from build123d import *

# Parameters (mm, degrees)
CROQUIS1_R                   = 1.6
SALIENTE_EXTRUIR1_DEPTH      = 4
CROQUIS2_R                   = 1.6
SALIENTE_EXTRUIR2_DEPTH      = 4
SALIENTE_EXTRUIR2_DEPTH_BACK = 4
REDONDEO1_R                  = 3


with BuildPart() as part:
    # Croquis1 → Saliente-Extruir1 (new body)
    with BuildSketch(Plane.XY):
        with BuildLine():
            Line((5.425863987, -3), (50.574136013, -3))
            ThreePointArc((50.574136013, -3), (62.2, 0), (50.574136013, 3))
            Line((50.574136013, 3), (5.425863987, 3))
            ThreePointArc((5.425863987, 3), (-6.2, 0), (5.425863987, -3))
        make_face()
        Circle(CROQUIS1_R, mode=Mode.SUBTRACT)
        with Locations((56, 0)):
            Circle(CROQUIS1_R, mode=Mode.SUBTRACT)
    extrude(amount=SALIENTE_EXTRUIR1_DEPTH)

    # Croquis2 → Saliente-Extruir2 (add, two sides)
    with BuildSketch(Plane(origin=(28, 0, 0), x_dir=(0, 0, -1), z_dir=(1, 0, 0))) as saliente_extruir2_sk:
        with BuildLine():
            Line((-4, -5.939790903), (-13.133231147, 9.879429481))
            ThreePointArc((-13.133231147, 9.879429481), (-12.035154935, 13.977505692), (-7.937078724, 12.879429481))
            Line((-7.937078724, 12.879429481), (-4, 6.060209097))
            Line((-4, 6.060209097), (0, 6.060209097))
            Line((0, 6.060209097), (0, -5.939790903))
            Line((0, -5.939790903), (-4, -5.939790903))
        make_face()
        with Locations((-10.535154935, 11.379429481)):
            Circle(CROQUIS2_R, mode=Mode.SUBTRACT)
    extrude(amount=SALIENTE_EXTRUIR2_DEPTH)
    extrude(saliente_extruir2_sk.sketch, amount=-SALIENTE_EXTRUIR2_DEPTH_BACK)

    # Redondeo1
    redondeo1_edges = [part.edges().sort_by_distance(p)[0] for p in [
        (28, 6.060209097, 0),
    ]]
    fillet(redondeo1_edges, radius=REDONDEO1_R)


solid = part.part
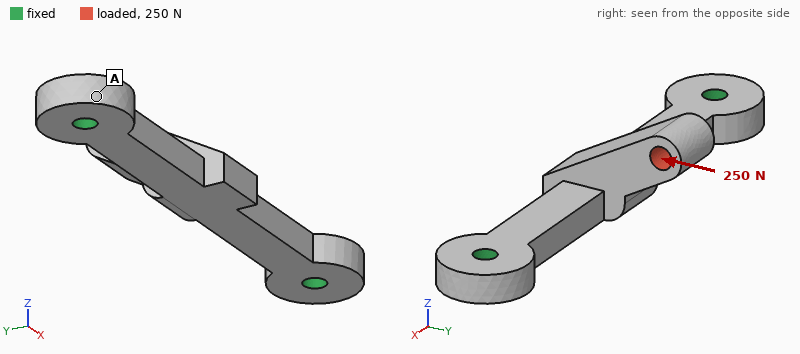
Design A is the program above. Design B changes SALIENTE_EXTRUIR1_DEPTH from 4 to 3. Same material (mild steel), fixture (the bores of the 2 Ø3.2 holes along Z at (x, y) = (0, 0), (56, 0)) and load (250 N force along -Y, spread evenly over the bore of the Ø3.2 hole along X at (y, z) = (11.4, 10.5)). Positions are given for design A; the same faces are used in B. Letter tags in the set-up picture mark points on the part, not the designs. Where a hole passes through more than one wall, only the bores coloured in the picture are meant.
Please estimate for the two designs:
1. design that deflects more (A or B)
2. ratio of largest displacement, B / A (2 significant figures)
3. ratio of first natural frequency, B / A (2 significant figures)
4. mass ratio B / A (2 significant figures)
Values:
B
2.0
0.70
0.84
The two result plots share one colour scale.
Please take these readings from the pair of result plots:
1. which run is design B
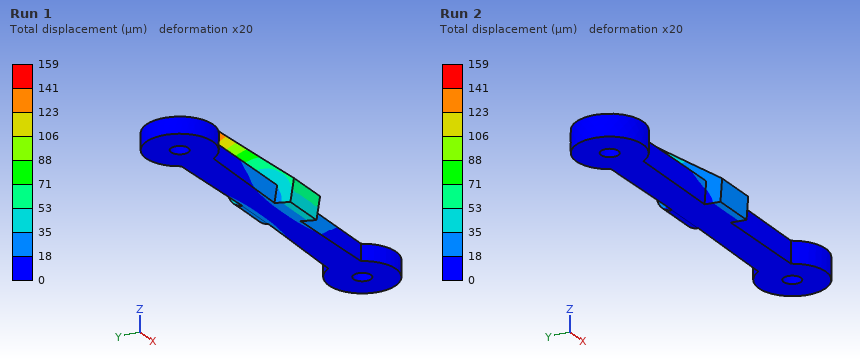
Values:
Run 1
